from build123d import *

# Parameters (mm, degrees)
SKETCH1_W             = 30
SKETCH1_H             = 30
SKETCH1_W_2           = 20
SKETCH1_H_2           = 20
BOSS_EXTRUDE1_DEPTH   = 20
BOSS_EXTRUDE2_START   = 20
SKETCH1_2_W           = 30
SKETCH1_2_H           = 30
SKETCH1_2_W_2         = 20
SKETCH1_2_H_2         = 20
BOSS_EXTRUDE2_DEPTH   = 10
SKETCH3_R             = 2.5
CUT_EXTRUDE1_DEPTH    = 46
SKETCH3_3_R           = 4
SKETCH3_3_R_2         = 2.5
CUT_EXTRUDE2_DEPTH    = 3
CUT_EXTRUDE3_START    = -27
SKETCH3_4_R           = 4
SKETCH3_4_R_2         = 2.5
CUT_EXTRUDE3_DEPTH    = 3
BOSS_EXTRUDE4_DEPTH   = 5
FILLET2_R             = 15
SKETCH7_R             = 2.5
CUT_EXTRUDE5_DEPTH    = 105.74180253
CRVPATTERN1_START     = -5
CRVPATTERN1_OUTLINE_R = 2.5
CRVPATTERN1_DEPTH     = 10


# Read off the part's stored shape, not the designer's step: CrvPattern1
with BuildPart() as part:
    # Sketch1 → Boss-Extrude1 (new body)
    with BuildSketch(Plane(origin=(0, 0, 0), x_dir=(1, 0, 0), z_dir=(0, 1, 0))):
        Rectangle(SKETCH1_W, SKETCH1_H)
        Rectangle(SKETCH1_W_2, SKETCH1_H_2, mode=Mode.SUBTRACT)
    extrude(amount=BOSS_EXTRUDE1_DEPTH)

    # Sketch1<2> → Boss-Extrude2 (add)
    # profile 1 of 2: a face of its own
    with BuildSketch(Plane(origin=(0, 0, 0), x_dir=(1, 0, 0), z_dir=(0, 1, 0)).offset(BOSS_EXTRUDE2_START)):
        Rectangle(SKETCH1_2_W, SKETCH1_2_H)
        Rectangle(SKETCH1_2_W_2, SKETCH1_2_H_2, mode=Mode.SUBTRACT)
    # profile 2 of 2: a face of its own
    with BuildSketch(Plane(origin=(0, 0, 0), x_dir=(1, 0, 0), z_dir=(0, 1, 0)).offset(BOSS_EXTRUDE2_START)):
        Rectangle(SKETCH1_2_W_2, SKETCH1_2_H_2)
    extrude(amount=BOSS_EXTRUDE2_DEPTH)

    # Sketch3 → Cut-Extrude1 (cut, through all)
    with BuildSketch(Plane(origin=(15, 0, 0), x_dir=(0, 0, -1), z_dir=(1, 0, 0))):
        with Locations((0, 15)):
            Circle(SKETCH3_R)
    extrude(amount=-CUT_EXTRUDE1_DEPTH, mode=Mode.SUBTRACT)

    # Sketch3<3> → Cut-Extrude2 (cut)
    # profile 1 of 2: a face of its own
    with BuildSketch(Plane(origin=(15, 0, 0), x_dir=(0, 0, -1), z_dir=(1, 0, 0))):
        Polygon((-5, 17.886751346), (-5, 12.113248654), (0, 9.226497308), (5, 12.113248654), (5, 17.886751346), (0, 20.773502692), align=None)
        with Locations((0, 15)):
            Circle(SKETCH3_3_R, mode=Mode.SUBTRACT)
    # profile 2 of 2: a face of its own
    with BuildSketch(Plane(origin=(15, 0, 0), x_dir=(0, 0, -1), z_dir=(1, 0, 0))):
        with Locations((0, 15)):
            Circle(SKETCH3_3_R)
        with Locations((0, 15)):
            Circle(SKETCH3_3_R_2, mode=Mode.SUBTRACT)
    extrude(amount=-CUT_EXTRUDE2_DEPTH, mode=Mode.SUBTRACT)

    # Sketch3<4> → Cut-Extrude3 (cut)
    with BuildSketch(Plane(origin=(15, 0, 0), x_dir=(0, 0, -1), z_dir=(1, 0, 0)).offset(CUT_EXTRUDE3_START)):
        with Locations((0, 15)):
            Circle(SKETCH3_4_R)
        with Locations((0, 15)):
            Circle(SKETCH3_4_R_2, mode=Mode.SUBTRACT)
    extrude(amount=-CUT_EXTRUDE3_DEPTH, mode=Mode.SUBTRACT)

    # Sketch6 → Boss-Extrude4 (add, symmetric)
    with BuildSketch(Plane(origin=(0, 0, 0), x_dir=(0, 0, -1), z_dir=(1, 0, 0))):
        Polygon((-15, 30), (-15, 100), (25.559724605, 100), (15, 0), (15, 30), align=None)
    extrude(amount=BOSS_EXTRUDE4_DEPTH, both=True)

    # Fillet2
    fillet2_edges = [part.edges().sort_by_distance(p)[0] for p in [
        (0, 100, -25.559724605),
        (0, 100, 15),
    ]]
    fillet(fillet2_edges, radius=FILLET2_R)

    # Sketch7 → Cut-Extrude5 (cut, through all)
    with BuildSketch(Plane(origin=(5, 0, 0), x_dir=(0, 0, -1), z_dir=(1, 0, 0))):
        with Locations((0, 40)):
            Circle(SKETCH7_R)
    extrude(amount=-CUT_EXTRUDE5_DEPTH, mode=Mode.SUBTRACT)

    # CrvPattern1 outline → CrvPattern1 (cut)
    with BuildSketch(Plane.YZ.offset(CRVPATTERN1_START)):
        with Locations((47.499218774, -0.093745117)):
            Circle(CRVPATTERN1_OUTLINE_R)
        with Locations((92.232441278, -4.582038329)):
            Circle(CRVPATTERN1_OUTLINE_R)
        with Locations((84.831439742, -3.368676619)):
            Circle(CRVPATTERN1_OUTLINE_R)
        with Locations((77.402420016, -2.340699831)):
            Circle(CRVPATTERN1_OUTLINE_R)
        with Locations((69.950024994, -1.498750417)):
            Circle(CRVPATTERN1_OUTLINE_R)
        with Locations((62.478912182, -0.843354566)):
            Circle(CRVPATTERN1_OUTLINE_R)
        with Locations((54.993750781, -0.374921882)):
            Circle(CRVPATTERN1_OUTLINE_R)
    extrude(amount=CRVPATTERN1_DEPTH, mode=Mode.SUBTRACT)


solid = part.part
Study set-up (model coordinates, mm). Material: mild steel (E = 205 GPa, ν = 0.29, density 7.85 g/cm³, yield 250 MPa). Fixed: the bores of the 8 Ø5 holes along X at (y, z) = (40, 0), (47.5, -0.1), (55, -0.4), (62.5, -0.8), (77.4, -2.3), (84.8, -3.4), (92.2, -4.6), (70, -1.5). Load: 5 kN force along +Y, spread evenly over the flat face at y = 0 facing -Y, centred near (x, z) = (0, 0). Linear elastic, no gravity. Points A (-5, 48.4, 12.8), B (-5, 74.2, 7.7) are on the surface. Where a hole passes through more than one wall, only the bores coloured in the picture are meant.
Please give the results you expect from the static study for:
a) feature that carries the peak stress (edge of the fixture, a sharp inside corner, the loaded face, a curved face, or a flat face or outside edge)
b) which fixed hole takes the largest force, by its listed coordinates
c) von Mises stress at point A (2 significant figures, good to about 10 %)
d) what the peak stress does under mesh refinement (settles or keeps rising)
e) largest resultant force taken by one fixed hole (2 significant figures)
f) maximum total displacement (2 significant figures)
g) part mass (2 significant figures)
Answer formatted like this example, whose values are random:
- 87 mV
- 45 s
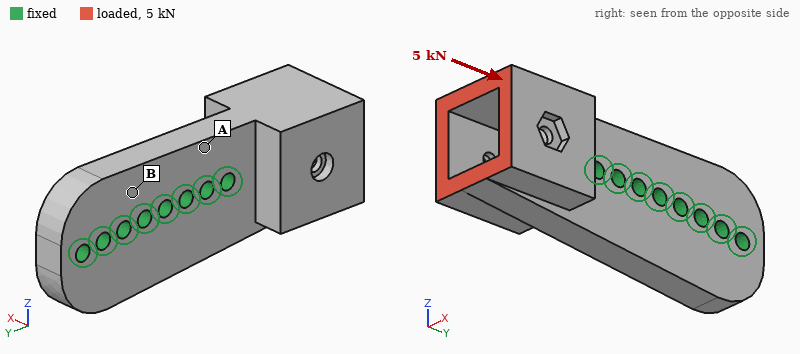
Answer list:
- edge of the fixture
- (40, 0)
- 8.1 MPa
- keeps rising
- 3.1 kN
- 4.0 µm
- 330 g
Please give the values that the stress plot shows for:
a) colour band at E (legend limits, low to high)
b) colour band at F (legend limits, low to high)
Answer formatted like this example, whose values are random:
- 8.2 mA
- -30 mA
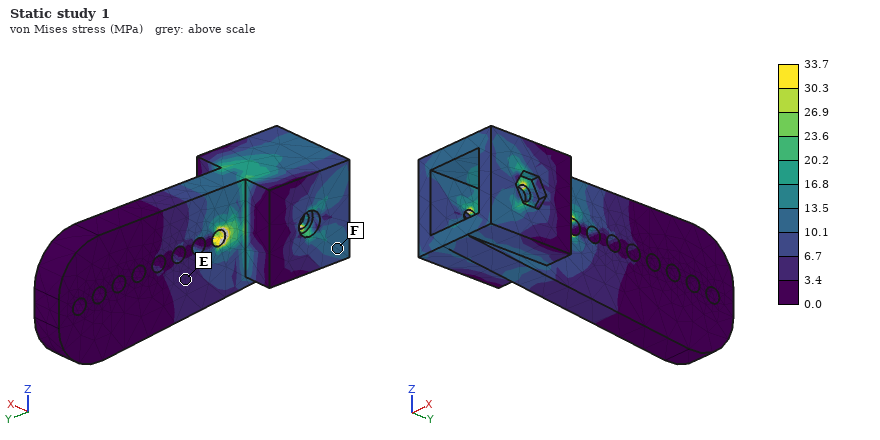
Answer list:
- 3.4 to 6.7 MPa
- 10.1 to 13.5 MPa
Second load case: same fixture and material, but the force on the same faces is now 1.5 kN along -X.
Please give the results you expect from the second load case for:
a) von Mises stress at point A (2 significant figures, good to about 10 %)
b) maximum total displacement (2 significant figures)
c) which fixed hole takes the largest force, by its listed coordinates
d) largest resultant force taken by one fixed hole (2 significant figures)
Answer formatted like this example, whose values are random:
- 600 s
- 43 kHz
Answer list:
- 22 MPa
- 57 µm
- (40, 0)
- 3.1 kN
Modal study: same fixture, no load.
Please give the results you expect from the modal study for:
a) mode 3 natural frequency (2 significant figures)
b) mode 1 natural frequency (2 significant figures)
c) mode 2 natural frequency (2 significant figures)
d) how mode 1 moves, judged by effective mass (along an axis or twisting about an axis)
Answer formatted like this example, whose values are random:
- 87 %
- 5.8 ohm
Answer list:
- 7200 Hz
- 3600 Hz
- 7000 Hz
- along X
